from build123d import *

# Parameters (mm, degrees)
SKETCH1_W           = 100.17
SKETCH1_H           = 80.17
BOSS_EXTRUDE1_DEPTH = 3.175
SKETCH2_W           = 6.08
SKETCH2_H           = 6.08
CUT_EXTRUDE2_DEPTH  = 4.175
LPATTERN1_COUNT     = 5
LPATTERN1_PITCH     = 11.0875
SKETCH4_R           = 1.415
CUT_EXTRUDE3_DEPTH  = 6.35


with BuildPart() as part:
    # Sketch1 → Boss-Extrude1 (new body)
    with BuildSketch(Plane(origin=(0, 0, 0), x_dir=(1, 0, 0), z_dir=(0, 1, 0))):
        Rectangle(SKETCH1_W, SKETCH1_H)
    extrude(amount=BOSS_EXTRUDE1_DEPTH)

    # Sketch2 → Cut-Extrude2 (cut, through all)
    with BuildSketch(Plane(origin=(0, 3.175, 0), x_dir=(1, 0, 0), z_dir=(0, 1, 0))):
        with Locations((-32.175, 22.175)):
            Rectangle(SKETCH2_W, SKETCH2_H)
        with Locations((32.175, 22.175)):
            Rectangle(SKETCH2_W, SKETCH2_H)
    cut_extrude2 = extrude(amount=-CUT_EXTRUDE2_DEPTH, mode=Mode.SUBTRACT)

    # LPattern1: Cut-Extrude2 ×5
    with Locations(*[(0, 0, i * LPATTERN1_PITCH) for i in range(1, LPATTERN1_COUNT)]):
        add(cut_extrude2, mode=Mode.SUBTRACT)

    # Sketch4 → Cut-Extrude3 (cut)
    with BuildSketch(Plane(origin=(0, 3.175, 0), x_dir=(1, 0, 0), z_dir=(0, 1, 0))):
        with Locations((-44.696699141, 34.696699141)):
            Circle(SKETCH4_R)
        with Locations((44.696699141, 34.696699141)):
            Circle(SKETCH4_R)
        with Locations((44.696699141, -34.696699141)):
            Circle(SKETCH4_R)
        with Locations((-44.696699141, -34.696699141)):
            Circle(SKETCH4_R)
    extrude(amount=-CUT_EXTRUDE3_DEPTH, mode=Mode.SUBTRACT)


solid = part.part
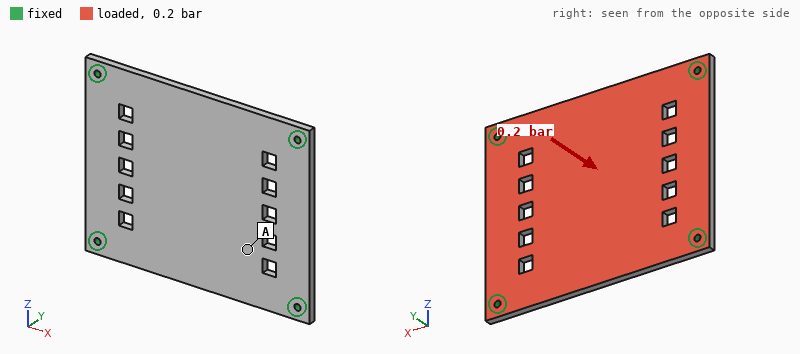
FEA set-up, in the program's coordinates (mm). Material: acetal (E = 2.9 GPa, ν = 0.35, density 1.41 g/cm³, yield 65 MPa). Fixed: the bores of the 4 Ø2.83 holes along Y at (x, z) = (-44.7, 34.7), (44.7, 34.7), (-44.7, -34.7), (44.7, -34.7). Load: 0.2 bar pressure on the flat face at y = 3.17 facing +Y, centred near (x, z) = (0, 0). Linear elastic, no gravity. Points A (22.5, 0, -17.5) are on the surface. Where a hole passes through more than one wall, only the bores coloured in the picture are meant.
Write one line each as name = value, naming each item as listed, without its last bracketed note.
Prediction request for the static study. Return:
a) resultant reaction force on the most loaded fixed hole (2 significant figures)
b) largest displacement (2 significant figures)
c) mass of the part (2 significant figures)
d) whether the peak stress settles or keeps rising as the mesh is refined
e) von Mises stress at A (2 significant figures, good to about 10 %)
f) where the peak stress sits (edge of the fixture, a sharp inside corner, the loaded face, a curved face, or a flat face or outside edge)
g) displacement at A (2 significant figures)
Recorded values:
resultant reaction force on the most loaded fixed hole = 38 N
largest displacement = 0.84 mm
mass of the part = 34 g
whether the peak stress settles or keeps rising as the mesh is refined = keeps rising
von Mises stress at A = 2.9 MPa
where the peak stress sits = edge of the fixture
displacement at A = 0.57 mm
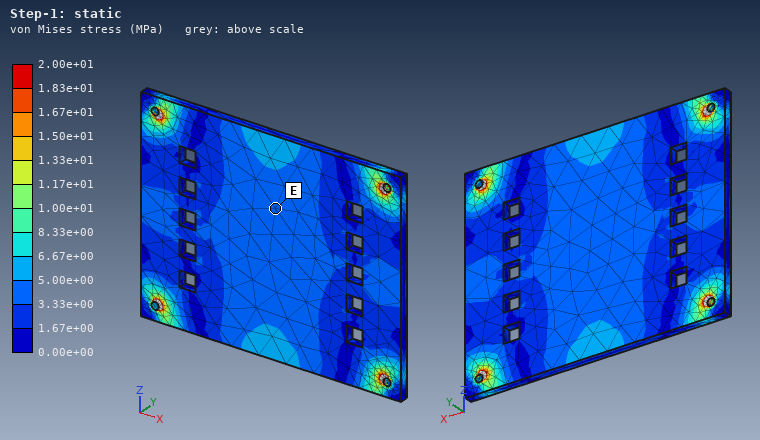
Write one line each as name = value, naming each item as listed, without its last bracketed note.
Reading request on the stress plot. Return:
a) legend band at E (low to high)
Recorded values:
legend band at E = 3.33e+00 to 5.00e+00 MPa
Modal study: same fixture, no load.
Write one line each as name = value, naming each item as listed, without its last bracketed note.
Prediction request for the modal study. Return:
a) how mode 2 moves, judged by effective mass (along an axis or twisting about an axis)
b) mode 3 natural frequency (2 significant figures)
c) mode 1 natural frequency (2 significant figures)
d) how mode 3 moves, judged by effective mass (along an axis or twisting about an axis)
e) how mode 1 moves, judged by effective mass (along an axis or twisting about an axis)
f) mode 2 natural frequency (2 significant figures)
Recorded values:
how mode 2 moves, judged by effective mass = twisting about X
mode 3 natural frequency = 910 Hz
mode 1 natural frequency = 430 Hz
how mode 3 moves, judged by effective mass = twisting about Z
how mode 1 moves, judged by effective mass = along Y
mode 2 natural frequency = 680 Hz
